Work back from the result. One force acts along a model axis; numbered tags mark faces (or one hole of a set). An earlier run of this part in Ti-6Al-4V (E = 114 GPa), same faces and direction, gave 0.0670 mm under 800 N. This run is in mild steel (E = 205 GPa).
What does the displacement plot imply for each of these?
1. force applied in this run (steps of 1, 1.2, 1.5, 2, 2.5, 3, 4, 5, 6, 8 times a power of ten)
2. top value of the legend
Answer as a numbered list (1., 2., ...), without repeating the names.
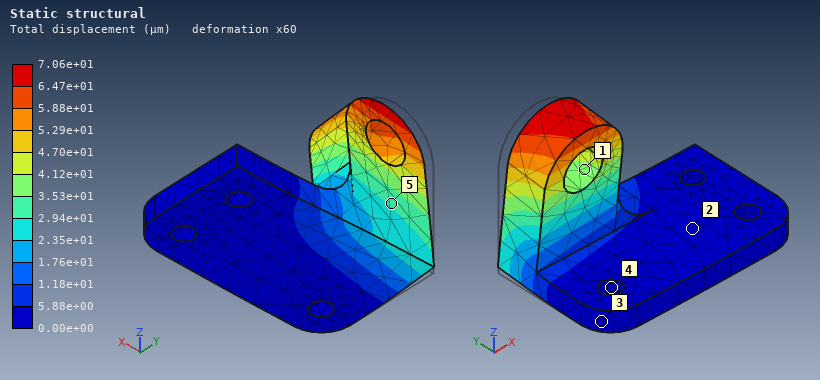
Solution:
1. 1.5 kN
2. 7.06e+01 µm
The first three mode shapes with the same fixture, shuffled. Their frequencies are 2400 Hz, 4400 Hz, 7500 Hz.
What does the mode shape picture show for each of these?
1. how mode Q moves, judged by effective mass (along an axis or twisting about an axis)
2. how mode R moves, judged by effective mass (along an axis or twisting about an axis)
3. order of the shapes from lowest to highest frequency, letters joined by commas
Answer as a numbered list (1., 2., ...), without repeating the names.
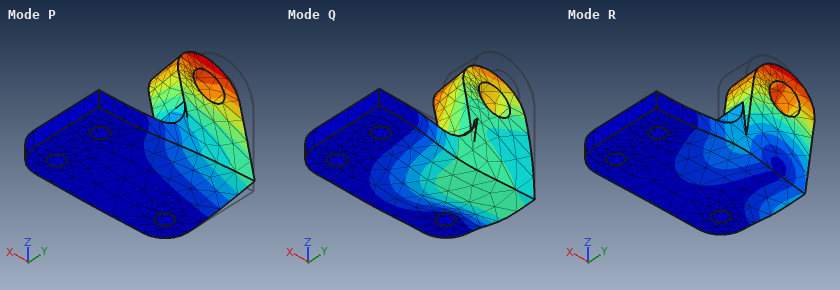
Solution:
1. along Z
2. along X
3. P, R, Q
